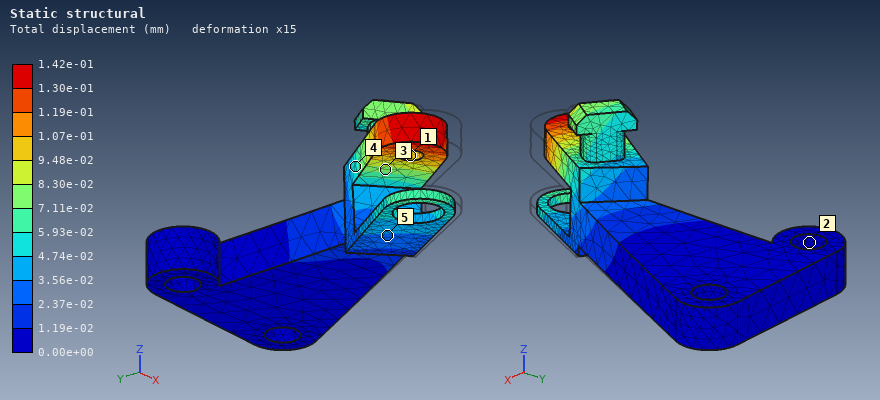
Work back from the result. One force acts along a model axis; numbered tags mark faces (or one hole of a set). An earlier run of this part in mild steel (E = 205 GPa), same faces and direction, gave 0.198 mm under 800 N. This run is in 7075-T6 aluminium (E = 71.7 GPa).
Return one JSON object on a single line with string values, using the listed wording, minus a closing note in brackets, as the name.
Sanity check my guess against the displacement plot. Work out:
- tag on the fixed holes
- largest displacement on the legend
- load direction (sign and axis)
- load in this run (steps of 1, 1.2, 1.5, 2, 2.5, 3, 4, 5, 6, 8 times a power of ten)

{"tag on the fixed holes": "2", "largest displacement on the legend": "1.42e-01 mm", "load direction": "-X", "load in this run": "200 N"}
